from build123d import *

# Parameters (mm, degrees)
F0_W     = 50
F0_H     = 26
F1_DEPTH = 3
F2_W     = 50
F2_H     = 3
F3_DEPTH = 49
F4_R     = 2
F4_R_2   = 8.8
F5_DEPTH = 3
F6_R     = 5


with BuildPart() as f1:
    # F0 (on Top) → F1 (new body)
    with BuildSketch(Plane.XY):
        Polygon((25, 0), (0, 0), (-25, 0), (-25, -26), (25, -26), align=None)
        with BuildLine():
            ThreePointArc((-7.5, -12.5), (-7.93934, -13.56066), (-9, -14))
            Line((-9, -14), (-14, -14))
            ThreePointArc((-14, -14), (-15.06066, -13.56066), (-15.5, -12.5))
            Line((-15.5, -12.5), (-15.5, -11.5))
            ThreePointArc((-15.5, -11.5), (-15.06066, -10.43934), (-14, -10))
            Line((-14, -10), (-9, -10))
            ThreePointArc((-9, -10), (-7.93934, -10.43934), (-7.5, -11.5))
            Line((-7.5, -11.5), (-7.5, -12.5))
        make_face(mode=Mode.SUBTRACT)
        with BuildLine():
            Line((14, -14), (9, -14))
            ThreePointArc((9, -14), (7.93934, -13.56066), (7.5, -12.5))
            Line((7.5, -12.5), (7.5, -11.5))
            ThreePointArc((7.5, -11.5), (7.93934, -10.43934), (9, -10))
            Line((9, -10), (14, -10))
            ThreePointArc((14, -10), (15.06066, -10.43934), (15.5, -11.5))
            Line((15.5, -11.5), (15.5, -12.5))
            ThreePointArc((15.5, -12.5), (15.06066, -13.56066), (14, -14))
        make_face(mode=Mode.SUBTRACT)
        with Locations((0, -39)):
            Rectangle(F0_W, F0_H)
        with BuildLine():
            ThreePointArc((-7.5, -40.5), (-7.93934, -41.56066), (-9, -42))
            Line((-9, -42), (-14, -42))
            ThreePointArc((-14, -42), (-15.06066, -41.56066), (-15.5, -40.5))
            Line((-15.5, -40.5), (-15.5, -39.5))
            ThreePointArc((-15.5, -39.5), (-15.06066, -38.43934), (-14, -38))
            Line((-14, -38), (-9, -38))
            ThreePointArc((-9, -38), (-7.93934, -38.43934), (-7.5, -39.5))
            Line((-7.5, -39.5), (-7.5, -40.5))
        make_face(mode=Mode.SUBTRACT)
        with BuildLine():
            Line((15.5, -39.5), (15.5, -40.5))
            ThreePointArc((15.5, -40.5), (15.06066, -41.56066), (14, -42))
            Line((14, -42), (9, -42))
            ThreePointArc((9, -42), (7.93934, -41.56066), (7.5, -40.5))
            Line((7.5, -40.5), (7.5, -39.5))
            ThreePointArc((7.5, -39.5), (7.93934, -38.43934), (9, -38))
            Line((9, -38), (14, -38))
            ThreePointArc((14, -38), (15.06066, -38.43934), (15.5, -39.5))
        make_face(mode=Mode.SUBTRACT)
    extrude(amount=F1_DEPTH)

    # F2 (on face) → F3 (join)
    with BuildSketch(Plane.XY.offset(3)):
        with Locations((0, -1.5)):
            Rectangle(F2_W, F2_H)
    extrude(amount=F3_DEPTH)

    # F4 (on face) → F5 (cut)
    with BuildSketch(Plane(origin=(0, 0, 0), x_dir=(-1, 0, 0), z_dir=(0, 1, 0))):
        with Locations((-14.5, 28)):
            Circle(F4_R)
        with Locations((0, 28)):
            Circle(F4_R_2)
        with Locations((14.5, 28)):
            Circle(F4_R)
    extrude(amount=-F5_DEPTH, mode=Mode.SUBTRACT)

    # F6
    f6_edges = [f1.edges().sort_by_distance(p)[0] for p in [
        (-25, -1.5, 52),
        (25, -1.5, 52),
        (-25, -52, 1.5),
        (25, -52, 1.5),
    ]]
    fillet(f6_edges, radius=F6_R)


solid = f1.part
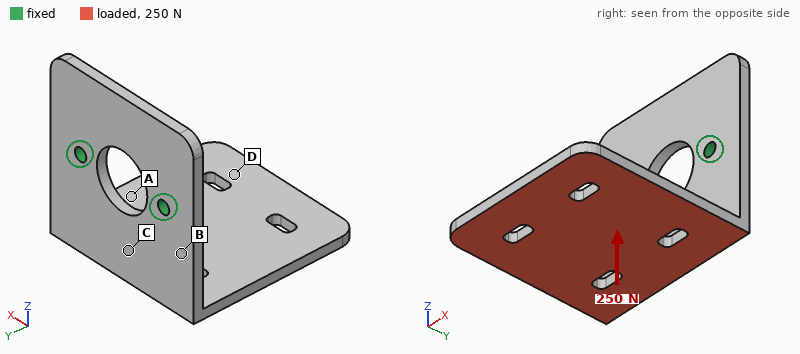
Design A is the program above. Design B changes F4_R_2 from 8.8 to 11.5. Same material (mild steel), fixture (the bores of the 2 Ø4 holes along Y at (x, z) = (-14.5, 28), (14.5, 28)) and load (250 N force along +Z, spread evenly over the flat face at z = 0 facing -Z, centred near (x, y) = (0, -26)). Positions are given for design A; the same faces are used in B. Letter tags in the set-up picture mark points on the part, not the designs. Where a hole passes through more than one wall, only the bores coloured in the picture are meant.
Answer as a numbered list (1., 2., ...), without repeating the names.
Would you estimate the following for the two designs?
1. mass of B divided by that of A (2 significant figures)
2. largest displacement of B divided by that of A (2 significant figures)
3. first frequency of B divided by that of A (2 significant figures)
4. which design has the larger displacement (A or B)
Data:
1. 0.96
2. 1.1
3. 0.94
4. B
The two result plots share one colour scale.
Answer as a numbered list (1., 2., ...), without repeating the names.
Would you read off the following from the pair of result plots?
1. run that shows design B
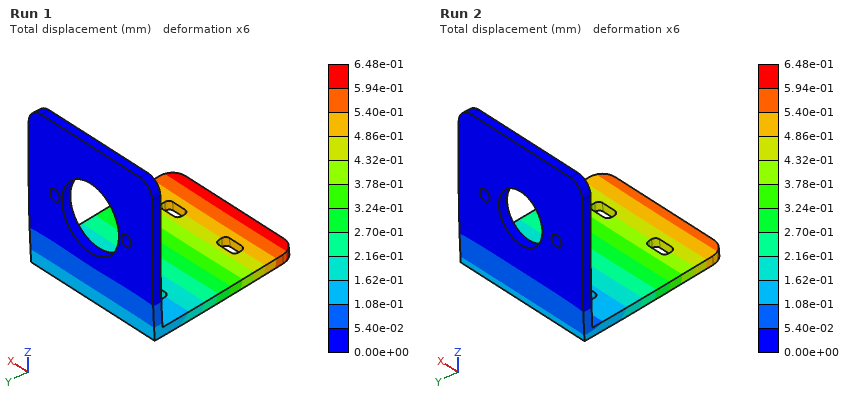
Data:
1. Run 1
